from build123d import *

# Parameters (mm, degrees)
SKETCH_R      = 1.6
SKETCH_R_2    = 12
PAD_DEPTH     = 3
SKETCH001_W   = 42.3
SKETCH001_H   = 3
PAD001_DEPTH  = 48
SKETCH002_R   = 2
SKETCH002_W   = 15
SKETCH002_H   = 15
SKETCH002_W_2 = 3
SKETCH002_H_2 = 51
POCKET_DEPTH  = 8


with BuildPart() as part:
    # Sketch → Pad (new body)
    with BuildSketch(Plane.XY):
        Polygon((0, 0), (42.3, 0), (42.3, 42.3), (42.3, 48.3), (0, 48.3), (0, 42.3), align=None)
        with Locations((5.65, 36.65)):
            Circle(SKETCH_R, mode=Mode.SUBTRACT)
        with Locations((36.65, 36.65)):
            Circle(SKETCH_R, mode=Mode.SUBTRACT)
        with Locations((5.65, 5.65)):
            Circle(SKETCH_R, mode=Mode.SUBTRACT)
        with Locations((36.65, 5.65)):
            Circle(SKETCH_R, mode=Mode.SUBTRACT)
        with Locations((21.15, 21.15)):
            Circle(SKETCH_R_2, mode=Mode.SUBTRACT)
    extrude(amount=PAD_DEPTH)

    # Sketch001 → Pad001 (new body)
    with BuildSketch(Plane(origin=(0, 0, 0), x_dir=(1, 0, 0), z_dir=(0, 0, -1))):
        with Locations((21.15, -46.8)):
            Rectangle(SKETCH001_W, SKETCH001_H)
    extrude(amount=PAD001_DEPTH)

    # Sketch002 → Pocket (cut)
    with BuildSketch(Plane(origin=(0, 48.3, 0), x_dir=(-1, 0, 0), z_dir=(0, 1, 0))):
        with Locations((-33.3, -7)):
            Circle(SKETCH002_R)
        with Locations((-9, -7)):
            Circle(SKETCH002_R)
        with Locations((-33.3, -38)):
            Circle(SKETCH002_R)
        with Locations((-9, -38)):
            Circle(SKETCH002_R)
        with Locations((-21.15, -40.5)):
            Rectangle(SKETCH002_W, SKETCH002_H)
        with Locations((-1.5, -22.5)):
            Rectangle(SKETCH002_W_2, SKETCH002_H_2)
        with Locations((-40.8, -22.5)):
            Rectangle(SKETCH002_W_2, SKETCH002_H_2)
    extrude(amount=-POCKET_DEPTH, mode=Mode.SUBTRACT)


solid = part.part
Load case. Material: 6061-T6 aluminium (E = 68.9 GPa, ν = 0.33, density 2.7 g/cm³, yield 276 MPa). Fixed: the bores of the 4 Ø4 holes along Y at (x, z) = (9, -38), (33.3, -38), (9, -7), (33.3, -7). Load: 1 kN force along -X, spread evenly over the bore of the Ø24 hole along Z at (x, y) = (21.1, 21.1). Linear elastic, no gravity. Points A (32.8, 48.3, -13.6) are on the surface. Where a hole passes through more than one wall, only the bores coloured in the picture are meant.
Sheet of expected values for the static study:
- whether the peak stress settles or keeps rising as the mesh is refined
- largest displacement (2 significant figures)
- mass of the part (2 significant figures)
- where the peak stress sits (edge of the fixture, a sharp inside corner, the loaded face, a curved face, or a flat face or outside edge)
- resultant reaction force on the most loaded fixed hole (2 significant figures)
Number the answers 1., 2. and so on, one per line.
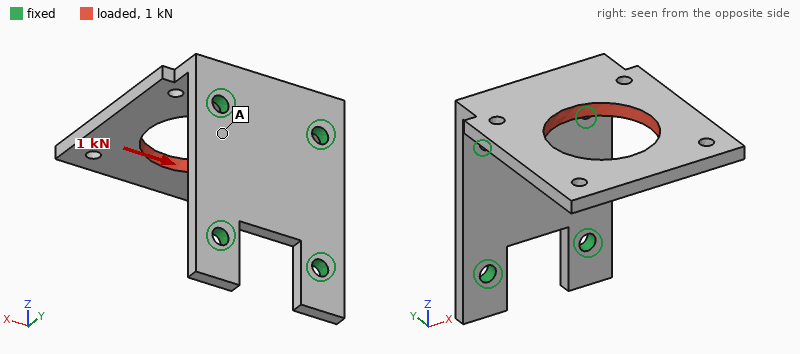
1. keeps rising
2. 0.29 mm
3. 24 g
4. edge of the fixture
5. 1.1 kN
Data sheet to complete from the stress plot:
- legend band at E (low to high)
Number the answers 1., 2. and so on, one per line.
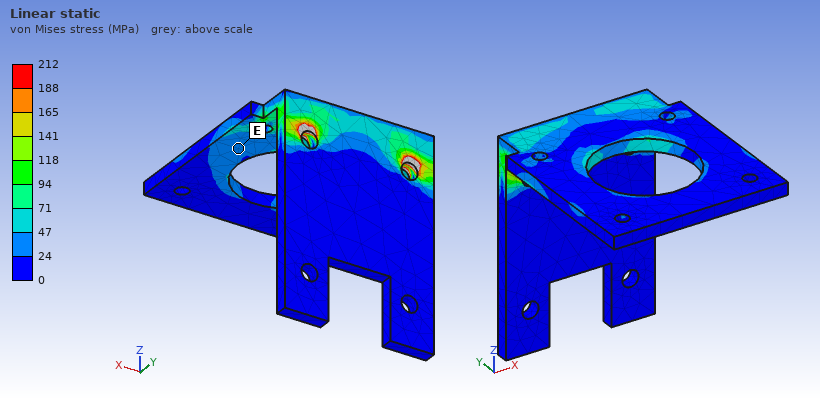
1. 24 to 47 MPa
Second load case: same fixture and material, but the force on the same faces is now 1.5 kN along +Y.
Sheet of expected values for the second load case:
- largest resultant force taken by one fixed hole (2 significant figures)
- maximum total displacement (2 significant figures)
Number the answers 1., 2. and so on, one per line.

1. 770 N
2. 0.41 mm
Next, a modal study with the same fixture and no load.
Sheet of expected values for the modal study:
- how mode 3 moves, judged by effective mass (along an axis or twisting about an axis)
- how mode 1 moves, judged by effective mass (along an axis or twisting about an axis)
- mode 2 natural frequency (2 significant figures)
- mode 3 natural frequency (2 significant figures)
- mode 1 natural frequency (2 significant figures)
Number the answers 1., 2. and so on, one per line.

1. along X
2. along Z
3. 2200 Hz
4. 3600 Hz
5. 860 Hz
